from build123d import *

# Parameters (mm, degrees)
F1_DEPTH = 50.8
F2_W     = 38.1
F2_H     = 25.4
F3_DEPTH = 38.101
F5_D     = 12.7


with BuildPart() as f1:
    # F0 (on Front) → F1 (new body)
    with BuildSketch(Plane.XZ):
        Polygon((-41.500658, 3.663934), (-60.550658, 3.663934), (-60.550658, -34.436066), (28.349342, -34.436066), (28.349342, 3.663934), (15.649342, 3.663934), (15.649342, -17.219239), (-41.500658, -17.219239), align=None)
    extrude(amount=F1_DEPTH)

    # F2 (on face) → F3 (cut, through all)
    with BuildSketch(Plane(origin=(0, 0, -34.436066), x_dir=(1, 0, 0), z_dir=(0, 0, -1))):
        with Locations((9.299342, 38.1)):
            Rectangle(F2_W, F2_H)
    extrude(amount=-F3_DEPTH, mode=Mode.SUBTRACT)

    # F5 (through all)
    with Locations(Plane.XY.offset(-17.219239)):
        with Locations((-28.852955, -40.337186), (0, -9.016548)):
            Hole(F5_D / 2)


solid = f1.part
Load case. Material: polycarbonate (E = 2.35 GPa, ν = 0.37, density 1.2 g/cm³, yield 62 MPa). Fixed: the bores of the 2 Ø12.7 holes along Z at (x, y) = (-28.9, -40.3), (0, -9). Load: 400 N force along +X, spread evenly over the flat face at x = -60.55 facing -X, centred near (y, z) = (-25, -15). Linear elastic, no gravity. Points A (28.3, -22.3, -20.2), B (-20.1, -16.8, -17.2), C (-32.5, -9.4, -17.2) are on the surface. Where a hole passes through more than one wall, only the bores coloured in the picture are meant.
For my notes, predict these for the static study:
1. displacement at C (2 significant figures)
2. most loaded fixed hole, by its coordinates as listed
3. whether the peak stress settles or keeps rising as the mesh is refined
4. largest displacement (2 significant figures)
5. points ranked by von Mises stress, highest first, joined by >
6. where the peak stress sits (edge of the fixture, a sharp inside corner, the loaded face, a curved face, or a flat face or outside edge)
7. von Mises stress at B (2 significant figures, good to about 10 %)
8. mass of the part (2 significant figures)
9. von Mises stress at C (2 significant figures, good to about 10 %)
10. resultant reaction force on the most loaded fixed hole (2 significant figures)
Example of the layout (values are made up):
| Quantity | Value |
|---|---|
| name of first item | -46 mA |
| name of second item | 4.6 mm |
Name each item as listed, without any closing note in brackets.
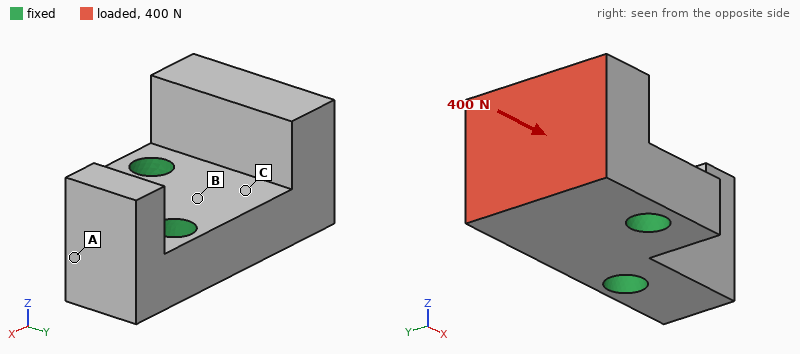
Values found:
| Quantity | Value |
|---|---|
| displacement at C | 14 µm |
| most loaded fixed hole, by its coordinates as listed | (-28.9, -40.3) |
| whether the peak stress settles or keeps rising as the mesh is refined | keeps rising |
| largest displacement | 83 µm |
| points ranked by von Mises stress, highest first, joined by > | C > B > A |
| where the peak stress sits | edge of the fixture |
| von Mises stress at B | 0.89 MPa |
| mass of the part | 100 g |
| von Mises stress at C | 1.4 MPa |
| resultant reaction force on the most loaded fixed hole | 230 N |
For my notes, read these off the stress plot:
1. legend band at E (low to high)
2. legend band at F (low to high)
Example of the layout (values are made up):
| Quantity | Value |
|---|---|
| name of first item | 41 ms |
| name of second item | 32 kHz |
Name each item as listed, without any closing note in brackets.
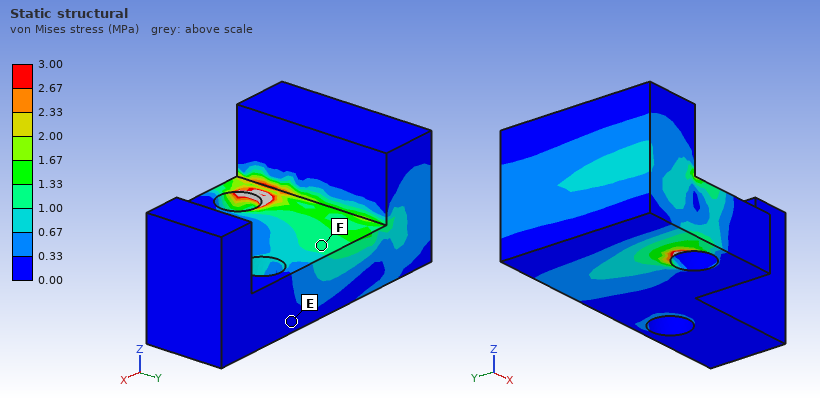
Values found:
| Quantity | Value |
|---|---|
| legend band at E | 0.00 to 0.33 MPa |
| legend band at F | 1.00 to 1.33 MPa |
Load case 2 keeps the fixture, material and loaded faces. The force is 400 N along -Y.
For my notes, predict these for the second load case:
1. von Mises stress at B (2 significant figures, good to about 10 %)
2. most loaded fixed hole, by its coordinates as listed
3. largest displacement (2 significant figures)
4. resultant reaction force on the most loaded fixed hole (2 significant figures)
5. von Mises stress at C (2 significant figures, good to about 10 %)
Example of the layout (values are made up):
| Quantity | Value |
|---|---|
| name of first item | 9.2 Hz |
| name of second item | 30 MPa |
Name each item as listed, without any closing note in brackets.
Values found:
| Quantity | Value |
|---|---|
| von Mises stress at B | 0.63 MPa |
| most loaded fixed hole, by its coordinates as listed | (-28.9, -40.3) |
| largest displacement | 74 µm |
| resultant reaction force on the most loaded fixed hole | 500 N |
| von Mises stress at C | 1.3 MPa |
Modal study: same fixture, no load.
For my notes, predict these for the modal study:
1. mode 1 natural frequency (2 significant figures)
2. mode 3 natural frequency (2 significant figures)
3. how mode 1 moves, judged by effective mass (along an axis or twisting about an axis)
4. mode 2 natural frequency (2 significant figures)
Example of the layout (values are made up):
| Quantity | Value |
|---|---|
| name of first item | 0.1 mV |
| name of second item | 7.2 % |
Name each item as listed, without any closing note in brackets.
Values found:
| Quantity | Value |
|---|---|
| mode 1 natural frequency | 1500 Hz |
| mode 3 natural frequency | 2300 Hz |
| how mode 1 moves, judged by effective mass | along Z |
| mode 2 natural frequency | 2200 Hz |
